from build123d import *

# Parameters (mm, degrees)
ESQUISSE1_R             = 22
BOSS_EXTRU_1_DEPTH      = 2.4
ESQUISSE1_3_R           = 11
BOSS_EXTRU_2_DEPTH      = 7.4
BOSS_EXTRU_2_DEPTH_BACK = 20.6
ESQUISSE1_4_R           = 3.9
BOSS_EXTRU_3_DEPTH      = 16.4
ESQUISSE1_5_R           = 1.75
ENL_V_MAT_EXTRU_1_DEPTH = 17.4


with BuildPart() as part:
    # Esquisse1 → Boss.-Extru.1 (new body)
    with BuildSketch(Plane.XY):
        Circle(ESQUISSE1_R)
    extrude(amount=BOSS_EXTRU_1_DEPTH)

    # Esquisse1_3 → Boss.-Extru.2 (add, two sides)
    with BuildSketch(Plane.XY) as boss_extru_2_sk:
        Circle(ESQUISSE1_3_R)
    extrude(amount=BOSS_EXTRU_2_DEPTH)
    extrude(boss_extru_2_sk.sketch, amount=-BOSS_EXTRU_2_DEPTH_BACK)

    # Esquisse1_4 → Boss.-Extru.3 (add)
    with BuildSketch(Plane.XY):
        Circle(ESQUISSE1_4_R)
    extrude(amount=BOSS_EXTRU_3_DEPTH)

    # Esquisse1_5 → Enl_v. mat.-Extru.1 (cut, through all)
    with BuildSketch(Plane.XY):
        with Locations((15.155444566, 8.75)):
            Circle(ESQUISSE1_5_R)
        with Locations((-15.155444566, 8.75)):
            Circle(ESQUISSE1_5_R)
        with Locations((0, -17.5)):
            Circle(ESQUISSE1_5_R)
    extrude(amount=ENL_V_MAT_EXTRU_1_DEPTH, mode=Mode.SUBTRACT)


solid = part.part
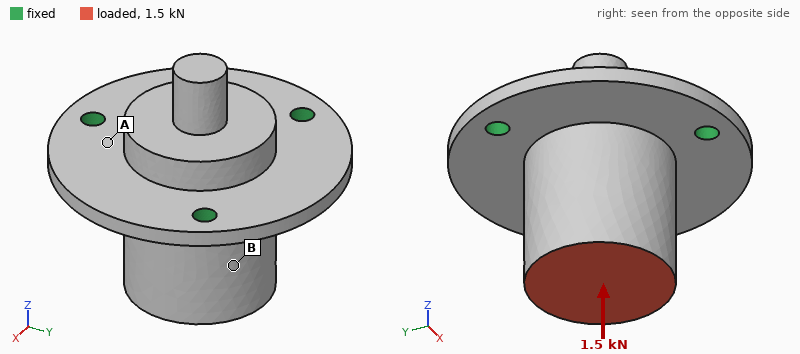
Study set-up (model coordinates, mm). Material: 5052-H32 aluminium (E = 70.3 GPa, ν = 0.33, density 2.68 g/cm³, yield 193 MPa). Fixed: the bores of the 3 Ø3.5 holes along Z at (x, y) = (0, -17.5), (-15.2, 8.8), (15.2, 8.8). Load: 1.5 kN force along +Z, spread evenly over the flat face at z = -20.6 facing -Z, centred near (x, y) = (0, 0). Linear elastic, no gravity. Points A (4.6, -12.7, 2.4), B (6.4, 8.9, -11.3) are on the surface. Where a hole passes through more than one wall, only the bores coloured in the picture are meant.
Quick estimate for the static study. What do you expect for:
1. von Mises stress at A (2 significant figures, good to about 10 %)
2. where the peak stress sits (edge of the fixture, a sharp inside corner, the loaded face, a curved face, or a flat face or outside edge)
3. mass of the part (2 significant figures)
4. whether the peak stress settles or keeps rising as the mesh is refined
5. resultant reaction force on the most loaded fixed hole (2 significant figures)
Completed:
26 MPa
edge of the fixture
37 g
keeps rising
500 N
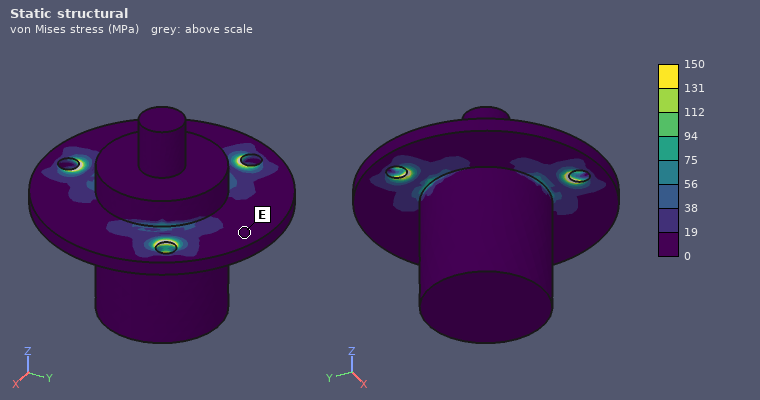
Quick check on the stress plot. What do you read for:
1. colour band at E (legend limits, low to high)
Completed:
0 to 19 MPa
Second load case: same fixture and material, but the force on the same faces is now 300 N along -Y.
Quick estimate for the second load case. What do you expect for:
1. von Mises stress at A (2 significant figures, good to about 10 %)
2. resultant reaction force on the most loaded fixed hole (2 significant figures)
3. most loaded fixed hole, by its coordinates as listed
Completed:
17 MPa
310 N
(0, -17.5)
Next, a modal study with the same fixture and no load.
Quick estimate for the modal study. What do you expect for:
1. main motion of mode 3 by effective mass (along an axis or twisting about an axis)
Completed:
along Z
